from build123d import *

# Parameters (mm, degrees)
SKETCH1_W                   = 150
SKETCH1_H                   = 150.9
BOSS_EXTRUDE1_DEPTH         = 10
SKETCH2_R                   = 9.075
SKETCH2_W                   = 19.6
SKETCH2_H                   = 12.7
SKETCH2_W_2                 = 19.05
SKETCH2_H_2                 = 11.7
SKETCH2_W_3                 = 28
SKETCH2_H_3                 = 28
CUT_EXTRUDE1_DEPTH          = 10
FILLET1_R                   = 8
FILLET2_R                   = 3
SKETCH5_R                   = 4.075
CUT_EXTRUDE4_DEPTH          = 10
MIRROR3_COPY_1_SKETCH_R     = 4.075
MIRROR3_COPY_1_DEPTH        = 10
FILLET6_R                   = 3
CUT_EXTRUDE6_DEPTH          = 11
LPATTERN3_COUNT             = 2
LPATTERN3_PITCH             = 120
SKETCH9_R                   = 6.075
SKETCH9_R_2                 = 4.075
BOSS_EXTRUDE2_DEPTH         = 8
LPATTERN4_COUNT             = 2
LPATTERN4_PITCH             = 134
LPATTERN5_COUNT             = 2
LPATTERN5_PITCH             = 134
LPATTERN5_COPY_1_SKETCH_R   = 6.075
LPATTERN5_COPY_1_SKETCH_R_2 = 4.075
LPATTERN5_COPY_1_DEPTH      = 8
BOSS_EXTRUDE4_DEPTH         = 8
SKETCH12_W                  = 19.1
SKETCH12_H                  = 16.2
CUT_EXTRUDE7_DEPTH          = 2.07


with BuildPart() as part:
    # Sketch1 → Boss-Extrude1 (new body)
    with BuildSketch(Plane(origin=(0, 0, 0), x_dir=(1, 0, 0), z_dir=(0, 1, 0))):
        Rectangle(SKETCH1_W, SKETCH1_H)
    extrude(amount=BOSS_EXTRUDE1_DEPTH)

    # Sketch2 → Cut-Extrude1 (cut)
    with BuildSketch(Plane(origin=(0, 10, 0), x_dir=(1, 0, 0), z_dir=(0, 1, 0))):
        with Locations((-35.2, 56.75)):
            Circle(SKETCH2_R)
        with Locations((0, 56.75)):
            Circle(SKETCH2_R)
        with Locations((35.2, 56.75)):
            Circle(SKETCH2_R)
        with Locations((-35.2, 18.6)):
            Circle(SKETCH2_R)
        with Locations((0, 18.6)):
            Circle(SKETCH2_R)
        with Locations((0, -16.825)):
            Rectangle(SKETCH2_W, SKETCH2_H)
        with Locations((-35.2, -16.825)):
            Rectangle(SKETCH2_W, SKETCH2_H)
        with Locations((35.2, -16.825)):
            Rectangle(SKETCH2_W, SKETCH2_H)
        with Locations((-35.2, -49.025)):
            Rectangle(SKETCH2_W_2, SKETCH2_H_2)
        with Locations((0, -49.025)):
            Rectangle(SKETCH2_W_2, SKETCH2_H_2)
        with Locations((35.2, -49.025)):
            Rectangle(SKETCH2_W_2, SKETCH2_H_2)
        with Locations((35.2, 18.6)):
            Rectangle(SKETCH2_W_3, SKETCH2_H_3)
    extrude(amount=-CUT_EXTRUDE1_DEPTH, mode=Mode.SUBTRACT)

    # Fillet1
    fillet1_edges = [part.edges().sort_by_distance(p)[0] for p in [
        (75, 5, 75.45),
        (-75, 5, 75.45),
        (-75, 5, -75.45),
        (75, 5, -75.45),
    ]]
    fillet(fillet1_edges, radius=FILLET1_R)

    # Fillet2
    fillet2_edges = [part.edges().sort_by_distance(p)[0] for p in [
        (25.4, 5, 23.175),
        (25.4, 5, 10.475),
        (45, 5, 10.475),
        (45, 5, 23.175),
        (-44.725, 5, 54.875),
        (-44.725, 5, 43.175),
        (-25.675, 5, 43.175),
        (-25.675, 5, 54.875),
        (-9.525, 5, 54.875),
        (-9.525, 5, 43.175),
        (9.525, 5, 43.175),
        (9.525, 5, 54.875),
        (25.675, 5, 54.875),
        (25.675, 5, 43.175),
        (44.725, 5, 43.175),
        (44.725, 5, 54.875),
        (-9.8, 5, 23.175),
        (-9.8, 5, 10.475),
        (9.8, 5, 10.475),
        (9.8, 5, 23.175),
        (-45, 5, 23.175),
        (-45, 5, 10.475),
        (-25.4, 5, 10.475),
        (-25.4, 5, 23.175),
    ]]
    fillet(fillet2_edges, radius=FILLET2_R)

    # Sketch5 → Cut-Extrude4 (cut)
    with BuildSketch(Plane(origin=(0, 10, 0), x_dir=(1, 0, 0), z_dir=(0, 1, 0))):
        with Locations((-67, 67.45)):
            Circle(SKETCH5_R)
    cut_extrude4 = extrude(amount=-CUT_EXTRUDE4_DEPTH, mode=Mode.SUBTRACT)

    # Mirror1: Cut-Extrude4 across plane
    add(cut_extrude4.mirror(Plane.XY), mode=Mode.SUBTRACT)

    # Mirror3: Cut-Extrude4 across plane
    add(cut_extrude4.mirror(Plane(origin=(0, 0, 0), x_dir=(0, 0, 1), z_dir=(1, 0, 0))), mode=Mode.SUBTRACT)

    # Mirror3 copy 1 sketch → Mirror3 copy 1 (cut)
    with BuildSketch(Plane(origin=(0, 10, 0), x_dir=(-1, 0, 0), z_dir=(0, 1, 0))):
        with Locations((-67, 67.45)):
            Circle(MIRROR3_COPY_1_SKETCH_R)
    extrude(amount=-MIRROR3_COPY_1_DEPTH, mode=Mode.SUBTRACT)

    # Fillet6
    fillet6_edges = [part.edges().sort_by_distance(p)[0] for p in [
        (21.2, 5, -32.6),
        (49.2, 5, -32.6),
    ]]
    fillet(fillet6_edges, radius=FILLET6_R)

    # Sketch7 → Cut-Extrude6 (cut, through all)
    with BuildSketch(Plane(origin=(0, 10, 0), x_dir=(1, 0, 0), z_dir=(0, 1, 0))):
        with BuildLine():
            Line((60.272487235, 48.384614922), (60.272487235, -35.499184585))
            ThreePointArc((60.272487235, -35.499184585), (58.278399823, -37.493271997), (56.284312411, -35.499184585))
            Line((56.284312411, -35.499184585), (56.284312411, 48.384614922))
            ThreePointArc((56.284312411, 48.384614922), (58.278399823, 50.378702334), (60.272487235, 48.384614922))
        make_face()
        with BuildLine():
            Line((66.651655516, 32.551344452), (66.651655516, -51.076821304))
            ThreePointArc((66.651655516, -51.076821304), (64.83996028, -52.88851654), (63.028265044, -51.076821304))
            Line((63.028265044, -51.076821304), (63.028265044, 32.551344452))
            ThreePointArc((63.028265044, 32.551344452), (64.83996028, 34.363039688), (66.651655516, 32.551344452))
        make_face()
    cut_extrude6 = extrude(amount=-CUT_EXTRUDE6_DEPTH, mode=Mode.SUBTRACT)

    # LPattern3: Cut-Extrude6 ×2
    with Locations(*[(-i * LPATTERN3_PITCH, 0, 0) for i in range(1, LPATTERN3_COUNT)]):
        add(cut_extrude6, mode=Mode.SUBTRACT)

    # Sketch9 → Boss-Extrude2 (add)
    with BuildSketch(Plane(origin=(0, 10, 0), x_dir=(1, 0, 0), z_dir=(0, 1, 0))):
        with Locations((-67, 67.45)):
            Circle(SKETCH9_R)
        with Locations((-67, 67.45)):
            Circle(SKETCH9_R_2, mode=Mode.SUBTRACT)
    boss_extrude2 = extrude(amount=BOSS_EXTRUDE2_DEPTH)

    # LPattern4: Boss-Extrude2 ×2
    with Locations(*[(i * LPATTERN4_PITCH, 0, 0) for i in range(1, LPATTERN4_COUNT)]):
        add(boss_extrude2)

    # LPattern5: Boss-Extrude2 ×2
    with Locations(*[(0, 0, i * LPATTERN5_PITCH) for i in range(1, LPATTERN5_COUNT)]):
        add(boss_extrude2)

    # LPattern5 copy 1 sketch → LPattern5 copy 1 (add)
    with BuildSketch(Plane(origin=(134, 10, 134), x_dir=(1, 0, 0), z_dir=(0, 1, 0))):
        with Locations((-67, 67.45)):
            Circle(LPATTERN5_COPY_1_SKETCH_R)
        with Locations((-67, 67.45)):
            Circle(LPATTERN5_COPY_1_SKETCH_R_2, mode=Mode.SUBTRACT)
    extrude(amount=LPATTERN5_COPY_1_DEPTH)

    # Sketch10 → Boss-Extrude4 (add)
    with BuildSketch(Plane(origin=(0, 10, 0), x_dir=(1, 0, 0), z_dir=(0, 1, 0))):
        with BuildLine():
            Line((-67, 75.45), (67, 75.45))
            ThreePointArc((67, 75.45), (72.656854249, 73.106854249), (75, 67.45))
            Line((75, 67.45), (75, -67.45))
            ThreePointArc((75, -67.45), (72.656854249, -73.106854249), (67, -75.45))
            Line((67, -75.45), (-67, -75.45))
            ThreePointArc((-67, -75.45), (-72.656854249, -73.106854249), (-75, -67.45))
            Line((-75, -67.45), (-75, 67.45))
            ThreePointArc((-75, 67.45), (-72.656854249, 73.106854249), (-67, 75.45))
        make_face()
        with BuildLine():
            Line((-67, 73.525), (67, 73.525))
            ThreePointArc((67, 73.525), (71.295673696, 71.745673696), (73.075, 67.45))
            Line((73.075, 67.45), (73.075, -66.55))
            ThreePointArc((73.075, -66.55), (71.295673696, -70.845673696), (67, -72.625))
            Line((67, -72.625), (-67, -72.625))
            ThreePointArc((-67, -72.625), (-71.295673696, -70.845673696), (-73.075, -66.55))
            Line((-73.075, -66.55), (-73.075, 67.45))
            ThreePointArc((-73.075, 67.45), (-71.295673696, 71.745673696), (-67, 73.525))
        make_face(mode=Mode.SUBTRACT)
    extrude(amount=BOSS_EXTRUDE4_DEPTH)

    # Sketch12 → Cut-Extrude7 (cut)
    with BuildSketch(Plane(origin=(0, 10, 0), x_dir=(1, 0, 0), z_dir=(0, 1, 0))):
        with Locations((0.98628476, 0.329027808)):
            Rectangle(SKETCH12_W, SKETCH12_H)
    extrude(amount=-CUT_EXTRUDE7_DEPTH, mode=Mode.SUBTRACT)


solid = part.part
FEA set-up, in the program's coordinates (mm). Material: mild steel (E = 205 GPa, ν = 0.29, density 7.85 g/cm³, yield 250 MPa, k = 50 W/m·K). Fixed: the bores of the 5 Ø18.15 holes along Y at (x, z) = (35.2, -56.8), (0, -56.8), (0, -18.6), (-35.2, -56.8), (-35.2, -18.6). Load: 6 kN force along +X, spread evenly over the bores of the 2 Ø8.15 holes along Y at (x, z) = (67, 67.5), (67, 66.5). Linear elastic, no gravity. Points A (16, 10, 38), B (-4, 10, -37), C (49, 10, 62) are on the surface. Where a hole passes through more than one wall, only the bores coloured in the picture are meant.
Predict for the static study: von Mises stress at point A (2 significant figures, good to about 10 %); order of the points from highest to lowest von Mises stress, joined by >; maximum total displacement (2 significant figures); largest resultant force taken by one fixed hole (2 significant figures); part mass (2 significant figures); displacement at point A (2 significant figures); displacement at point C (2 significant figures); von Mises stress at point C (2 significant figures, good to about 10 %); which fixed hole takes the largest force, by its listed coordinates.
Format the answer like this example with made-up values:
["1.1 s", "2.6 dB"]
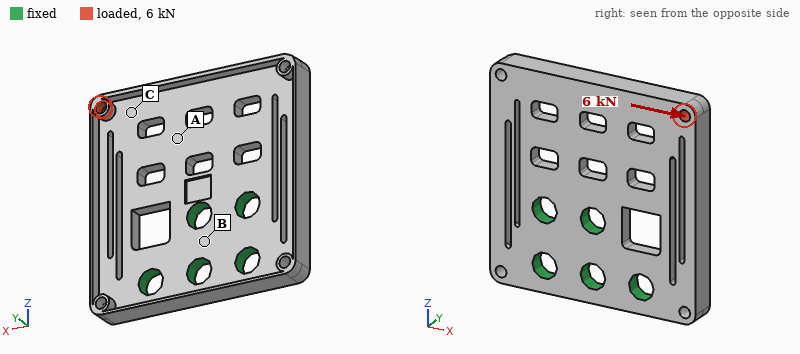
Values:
["19 MPa", "C > A > B", "0.10 mm", "6.0 kN", "1.5 kg", "0.020 mm", "0.055 mm", "37 MPa", "(-35.2, -18.6)"]
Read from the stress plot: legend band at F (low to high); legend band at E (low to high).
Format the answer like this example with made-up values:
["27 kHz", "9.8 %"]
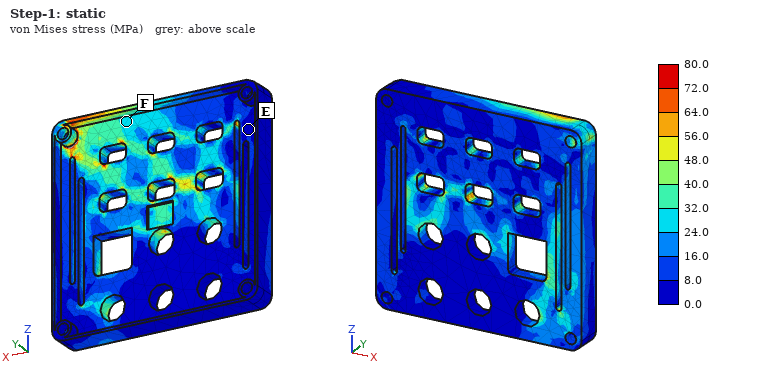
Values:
["24.0 to 32.0 MPa", "0.0 to 8.0 MPa"]
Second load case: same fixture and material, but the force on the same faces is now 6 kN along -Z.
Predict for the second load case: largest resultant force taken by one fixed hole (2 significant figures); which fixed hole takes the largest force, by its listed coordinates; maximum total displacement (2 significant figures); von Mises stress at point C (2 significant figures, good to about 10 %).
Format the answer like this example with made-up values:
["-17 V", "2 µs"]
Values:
["5.3 kN", "(35.2, -56.8)", "0.11 mm", "27 MPa"]
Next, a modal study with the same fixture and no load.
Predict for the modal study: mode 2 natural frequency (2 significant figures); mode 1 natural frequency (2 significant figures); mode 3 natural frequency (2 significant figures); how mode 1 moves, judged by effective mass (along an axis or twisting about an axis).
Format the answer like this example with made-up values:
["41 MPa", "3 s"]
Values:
["1100 Hz", "710 Hz", "2500 Hz", "along Y"]
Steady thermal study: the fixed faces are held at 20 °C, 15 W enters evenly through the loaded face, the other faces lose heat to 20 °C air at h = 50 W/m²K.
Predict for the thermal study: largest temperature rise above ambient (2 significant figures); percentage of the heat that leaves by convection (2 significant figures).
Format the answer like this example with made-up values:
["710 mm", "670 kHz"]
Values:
["38 K", "82 %"]
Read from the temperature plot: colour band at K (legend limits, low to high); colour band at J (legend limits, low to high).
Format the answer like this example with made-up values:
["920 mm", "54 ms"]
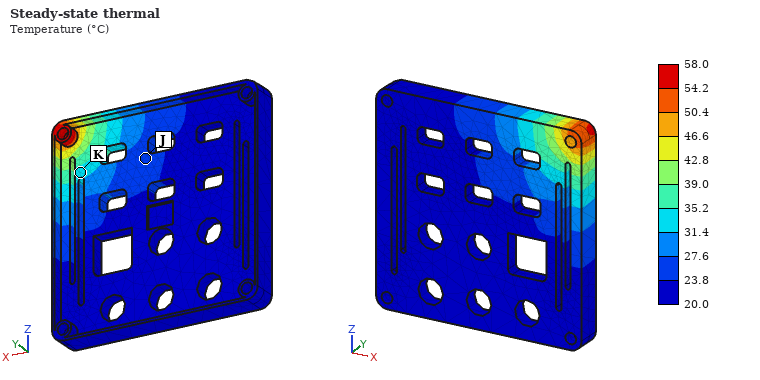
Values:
["31.4 to 35.2 °C", "23.8 to 27.6 °C"]
